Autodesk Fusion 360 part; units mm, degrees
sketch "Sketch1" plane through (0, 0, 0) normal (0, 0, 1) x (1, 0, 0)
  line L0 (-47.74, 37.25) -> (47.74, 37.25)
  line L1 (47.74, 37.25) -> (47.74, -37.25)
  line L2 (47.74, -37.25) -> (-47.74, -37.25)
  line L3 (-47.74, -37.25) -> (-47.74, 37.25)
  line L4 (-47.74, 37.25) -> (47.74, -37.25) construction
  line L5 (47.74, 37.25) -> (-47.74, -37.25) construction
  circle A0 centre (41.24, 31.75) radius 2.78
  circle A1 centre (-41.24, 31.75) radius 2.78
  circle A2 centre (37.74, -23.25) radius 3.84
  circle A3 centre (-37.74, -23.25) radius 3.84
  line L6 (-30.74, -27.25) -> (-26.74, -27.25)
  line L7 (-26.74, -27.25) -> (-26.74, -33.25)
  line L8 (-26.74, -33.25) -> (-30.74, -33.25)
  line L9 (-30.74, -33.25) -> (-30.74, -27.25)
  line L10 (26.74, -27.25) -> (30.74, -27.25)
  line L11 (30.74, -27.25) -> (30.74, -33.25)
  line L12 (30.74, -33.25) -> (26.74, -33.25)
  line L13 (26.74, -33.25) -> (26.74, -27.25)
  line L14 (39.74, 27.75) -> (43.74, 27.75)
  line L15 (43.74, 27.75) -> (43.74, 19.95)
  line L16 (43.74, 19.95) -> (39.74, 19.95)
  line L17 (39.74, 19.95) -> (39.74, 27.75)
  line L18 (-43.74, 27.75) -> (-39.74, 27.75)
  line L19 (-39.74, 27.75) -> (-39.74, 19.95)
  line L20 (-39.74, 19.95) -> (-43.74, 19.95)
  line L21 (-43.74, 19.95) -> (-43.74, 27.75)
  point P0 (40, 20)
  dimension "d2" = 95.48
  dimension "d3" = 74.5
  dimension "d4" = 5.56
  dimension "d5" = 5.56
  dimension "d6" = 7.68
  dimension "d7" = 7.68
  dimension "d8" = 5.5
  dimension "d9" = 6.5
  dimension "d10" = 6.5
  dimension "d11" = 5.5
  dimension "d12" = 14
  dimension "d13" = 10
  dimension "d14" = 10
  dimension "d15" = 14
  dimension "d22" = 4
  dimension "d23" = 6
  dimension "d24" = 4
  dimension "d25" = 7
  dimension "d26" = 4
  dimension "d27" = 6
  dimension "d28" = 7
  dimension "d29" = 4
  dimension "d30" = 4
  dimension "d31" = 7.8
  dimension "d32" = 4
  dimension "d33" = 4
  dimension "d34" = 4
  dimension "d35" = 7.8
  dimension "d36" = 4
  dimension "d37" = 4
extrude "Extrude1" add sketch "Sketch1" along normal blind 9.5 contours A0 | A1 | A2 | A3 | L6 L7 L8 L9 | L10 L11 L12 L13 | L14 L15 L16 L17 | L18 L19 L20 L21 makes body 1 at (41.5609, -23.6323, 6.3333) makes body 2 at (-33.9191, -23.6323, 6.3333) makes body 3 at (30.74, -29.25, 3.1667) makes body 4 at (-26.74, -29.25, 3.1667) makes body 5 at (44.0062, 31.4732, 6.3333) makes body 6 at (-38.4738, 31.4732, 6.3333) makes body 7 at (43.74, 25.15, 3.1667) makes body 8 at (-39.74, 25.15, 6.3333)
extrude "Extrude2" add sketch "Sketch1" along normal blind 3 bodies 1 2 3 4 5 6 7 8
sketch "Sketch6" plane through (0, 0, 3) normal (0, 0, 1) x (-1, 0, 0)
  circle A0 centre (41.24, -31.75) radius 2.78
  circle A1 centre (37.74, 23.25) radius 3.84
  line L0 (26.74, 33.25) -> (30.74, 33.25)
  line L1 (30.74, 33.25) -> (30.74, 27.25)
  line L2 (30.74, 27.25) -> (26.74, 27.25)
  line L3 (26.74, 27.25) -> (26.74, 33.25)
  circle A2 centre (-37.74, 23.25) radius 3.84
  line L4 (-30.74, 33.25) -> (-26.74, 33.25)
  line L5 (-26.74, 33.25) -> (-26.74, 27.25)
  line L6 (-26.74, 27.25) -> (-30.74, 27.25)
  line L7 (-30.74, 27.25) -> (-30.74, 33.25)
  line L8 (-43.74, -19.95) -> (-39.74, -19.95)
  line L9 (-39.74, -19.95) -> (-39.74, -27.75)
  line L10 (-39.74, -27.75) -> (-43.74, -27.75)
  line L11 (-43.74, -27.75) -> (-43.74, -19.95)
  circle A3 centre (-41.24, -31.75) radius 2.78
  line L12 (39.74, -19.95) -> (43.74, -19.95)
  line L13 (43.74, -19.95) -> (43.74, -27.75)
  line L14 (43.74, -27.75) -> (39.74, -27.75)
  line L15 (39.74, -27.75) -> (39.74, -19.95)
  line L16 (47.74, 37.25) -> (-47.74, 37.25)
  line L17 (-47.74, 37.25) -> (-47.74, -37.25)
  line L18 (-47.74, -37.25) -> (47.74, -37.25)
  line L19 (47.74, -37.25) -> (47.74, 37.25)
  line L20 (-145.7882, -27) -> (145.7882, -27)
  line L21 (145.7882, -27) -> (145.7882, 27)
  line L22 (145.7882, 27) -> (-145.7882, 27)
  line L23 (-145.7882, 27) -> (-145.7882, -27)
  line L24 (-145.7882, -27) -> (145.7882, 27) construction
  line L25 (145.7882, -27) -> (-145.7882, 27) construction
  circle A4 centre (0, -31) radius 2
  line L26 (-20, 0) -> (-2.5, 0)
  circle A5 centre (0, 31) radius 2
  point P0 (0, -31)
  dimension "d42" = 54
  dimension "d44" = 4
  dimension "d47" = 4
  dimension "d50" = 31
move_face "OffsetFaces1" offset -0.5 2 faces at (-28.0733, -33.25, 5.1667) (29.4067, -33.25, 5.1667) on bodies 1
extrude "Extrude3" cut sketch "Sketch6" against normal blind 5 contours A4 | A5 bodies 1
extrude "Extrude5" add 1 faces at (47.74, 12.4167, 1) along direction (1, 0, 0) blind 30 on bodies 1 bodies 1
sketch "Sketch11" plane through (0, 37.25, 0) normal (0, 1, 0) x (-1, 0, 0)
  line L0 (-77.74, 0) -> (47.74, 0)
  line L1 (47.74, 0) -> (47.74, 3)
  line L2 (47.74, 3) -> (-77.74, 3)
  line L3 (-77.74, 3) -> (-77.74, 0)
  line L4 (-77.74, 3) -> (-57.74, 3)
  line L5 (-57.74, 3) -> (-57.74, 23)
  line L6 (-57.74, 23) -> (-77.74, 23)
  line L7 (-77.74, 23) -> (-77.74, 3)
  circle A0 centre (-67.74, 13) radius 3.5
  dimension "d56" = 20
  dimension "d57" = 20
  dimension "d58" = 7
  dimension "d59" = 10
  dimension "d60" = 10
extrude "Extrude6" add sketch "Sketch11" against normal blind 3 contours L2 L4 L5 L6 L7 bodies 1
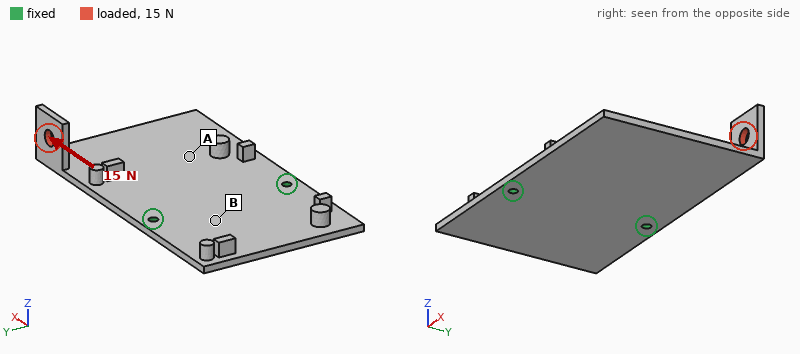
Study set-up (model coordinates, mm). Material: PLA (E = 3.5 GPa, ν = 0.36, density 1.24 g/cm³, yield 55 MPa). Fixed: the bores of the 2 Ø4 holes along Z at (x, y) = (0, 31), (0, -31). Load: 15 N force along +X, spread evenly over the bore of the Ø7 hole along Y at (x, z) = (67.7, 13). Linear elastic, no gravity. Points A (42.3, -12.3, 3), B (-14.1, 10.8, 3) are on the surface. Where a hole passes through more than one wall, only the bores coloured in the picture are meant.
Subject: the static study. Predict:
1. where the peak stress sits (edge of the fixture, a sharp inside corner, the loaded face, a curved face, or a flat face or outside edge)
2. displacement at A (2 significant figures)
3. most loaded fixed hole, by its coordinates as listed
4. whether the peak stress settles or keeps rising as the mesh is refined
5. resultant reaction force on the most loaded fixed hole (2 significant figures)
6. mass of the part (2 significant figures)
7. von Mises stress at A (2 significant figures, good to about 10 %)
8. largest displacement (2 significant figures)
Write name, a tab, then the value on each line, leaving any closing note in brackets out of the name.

where the peak stress sits	a sharp inside corner
displacement at A	0.32 mm
most loaded fixed hole, by its coordinates as listed	(0, 31)
whether the peak stress settles or keeps rising as the mesh is refined	keeps rising
resultant reaction force on the most loaded fixed hole	16 N
mass of the part	38 g
von Mises stress at A	1.2 MPa
largest displacement	1.4 mm
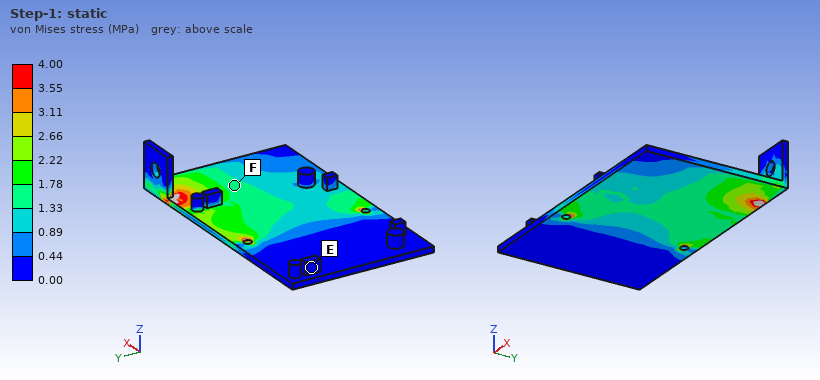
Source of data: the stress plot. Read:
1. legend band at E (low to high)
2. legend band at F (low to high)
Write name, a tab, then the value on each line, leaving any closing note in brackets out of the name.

legend band at E	0.00 to 0.44 MPa
legend band at F	1.33 to 1.78 MPa
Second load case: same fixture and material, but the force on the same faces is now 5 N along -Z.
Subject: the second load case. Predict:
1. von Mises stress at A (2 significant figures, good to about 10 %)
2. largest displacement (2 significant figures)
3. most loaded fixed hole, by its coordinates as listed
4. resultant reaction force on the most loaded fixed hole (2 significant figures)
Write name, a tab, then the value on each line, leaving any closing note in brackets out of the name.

von Mises stress at A	1.3 MPa
largest displacement	1.7 mm
most loaded fixed hole, by its coordinates as listed	(0, 31)
resultant reaction force on the most loaded fixed hole	5.5 N
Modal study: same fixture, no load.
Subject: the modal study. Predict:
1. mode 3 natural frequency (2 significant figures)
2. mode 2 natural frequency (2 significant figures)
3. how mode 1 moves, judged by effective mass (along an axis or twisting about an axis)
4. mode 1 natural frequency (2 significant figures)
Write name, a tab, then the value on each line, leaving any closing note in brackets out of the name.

mode 3 natural frequency	300 Hz
mode 2 natural frequency	290 Hz
how mode 1 moves, judged by effective mass	along Z
mode 1 natural frequency	110 Hz
